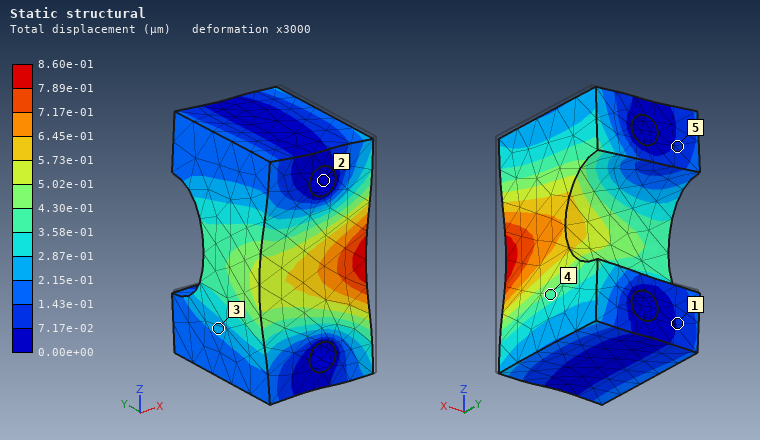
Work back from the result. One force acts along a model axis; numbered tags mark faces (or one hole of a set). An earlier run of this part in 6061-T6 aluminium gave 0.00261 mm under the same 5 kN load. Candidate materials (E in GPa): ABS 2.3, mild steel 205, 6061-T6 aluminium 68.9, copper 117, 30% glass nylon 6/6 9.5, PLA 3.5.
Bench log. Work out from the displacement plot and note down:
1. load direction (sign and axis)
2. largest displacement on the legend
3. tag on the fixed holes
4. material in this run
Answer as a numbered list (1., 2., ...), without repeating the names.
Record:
1. -X
2. 8.60e-01 µm
3. 2
4. mild steel
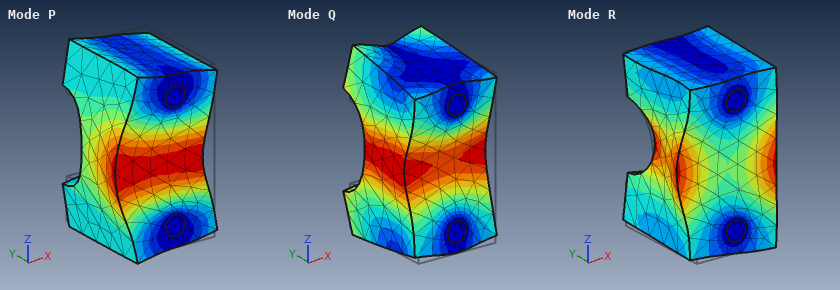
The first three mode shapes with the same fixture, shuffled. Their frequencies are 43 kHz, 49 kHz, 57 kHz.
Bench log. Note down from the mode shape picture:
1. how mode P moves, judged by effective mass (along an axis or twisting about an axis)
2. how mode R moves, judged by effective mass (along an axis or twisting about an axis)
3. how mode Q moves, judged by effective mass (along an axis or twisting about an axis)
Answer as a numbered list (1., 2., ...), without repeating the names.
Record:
1. along X
2. twisting about Z
3. along Y
